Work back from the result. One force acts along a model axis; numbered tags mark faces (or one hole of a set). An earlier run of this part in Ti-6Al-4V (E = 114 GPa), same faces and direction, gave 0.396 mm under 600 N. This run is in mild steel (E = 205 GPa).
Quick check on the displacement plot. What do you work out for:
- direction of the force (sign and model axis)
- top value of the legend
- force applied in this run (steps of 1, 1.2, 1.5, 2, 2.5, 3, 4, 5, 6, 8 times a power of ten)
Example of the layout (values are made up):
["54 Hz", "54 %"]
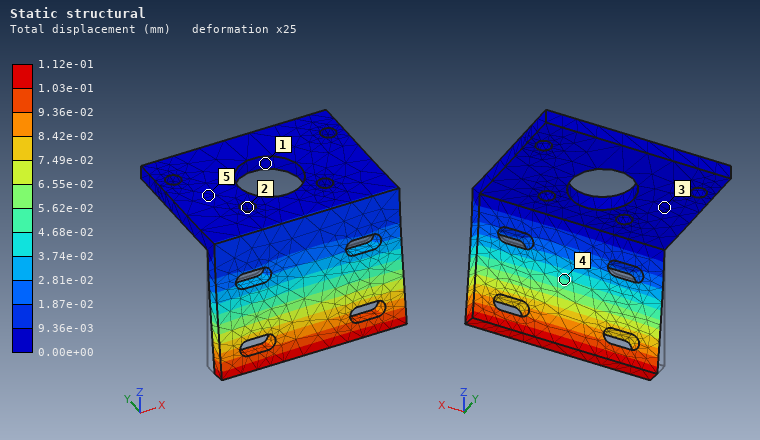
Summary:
["-Y", "1.12e-01 mm", "300 N"]
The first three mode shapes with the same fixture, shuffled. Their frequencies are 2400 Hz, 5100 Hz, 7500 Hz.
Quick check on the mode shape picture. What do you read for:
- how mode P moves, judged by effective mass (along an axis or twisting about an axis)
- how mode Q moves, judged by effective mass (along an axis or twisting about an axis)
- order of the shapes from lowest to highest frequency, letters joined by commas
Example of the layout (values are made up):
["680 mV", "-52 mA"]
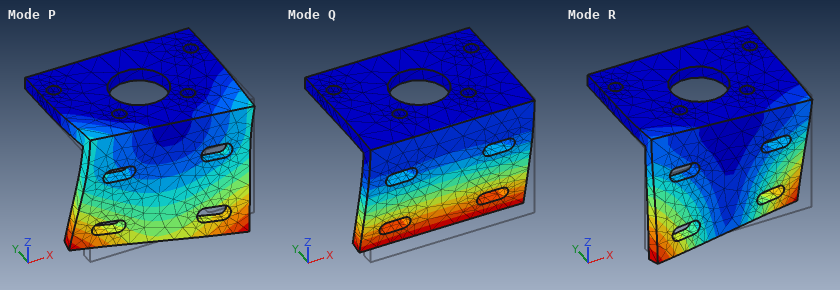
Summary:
["along X", "along Y", "Q, R, P"]
